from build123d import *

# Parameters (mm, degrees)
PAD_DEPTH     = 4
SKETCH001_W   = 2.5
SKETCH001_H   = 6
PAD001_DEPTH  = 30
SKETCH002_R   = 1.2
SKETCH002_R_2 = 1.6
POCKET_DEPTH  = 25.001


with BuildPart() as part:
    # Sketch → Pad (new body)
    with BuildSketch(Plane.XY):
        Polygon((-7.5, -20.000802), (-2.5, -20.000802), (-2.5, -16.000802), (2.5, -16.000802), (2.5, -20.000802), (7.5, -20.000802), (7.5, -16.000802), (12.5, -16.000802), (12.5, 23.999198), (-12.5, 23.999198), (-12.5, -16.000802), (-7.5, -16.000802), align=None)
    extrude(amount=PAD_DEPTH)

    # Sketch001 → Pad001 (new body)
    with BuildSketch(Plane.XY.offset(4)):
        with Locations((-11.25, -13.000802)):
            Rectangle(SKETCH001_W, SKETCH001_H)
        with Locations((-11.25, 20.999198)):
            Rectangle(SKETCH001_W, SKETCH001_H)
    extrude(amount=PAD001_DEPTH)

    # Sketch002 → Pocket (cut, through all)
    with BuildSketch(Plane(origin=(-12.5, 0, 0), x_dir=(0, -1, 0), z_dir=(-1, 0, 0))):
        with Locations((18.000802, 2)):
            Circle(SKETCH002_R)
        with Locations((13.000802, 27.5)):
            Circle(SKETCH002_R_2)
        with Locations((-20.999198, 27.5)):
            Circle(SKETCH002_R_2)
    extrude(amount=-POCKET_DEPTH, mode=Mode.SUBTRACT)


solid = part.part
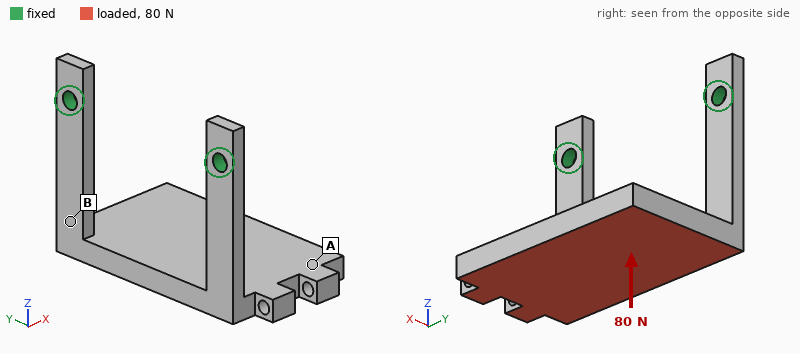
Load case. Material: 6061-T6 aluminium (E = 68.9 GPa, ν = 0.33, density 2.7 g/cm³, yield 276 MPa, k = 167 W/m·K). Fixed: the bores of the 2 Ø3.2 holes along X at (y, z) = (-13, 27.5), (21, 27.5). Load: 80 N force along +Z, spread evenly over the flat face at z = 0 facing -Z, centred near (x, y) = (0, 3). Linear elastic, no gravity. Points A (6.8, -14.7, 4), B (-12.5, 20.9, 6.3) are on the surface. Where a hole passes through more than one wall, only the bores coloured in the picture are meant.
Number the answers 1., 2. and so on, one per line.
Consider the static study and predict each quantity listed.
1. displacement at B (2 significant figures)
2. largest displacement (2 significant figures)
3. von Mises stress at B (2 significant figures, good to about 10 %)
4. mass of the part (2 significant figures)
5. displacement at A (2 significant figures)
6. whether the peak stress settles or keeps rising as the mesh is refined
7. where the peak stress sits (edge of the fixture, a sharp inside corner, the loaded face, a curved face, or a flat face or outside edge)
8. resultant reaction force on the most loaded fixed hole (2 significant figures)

1. 0.17 mm
2. 0.56 mm
3. 67 MPa
4. 13 g
5. 0.42 mm
6. keeps rising
7. edge of the fixture
8. 42 N
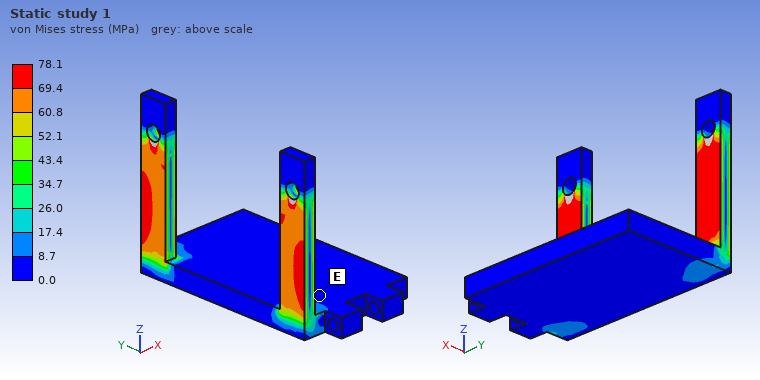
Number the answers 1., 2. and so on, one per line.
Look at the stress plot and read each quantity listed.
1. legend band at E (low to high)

1. 0.0 to 8.7 MPa
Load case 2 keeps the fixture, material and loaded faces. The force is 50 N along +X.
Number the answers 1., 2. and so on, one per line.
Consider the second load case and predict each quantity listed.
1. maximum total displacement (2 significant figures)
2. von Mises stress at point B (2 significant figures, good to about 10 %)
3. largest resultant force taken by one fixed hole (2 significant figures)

1. 0.48 mm
2. 26 MPa
3. 26 N
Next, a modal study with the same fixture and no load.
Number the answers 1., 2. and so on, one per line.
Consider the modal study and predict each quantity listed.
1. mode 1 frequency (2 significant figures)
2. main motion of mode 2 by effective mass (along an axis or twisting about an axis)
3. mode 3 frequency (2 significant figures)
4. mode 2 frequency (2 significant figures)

1. 530 Hz
2. along Y
3. 2000 Hz
4. 1300 Hz
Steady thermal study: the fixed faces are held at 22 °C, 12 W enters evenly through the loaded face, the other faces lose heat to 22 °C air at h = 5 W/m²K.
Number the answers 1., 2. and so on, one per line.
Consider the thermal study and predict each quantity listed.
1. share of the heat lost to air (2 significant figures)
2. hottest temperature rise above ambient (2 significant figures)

1. 4.9 %
2. 62 K
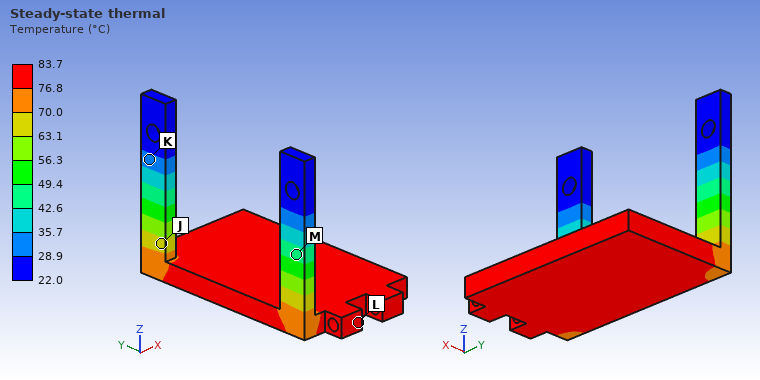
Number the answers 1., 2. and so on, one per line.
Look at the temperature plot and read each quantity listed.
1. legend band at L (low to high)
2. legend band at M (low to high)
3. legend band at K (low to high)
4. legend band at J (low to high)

1. 76.8 to 83.7 °C
2. 42.6 to 49.4 °C
3. 28.9 to 35.7 °C
4. 63.1 to 70.0 °C
